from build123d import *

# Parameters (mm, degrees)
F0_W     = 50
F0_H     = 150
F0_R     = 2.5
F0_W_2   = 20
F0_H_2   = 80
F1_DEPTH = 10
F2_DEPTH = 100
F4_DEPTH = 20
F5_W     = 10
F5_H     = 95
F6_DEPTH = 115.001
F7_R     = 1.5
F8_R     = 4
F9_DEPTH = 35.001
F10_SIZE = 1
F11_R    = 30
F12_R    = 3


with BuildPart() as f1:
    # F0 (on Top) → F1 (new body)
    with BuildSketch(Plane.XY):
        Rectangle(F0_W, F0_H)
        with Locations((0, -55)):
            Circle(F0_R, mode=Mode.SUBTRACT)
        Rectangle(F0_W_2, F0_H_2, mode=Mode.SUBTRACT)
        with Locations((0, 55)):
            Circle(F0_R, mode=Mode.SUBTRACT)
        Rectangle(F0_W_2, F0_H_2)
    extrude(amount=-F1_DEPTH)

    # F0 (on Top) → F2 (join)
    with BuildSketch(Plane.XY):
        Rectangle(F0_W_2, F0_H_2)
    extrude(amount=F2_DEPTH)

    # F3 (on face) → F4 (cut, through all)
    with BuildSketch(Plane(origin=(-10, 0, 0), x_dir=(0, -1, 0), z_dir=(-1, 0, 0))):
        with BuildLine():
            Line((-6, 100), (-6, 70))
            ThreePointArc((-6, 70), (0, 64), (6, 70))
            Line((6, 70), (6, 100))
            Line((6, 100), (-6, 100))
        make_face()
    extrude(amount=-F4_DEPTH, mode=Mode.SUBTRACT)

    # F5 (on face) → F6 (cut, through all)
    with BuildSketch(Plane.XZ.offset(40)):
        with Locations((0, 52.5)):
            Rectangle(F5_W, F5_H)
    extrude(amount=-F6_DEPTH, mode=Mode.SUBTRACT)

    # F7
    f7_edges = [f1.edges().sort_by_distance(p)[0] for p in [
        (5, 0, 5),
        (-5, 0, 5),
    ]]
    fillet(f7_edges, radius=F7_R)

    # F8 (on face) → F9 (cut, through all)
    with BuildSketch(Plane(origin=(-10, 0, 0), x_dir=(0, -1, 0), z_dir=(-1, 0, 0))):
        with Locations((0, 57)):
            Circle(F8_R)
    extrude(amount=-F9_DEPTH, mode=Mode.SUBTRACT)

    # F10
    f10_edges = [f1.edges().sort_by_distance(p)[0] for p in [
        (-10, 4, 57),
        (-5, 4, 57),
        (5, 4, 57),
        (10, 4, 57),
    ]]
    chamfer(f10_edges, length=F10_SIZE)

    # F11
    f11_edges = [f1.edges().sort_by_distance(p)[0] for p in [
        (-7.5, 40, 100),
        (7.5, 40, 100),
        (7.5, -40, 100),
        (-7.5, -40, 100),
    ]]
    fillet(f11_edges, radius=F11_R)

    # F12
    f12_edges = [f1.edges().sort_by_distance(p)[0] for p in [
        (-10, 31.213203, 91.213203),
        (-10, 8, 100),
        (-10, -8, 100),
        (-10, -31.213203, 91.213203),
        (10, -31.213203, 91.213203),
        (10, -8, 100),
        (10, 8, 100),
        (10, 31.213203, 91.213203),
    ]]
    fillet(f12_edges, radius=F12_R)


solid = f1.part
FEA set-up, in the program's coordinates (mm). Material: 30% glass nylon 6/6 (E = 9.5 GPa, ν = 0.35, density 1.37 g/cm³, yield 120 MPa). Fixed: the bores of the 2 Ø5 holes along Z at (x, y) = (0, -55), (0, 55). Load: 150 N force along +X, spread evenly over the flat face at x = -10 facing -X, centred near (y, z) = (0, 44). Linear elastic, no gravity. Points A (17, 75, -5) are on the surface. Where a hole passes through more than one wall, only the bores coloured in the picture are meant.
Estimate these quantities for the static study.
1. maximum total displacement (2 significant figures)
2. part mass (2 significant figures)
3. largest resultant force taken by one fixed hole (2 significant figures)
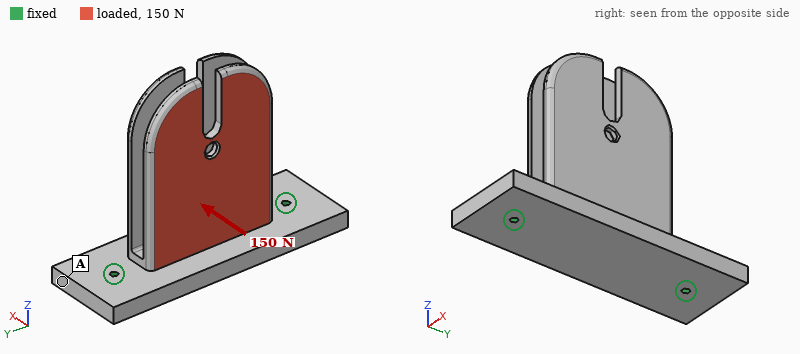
1.9 mm
200 g
76 N
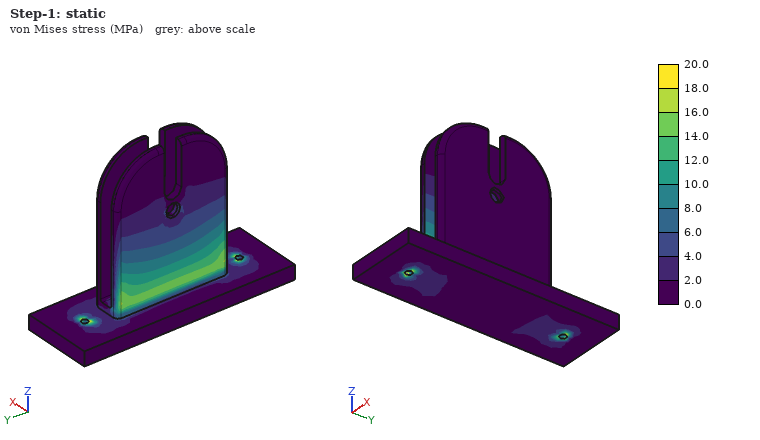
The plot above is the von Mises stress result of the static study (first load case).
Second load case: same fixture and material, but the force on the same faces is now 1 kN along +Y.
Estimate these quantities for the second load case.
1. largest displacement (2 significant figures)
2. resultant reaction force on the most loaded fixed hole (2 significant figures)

0.26 mm
730 N
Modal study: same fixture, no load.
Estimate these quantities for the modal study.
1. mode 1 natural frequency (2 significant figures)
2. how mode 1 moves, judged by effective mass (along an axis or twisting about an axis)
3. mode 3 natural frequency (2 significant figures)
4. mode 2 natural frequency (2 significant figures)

250 Hz
along X
580 Hz
280 Hz
